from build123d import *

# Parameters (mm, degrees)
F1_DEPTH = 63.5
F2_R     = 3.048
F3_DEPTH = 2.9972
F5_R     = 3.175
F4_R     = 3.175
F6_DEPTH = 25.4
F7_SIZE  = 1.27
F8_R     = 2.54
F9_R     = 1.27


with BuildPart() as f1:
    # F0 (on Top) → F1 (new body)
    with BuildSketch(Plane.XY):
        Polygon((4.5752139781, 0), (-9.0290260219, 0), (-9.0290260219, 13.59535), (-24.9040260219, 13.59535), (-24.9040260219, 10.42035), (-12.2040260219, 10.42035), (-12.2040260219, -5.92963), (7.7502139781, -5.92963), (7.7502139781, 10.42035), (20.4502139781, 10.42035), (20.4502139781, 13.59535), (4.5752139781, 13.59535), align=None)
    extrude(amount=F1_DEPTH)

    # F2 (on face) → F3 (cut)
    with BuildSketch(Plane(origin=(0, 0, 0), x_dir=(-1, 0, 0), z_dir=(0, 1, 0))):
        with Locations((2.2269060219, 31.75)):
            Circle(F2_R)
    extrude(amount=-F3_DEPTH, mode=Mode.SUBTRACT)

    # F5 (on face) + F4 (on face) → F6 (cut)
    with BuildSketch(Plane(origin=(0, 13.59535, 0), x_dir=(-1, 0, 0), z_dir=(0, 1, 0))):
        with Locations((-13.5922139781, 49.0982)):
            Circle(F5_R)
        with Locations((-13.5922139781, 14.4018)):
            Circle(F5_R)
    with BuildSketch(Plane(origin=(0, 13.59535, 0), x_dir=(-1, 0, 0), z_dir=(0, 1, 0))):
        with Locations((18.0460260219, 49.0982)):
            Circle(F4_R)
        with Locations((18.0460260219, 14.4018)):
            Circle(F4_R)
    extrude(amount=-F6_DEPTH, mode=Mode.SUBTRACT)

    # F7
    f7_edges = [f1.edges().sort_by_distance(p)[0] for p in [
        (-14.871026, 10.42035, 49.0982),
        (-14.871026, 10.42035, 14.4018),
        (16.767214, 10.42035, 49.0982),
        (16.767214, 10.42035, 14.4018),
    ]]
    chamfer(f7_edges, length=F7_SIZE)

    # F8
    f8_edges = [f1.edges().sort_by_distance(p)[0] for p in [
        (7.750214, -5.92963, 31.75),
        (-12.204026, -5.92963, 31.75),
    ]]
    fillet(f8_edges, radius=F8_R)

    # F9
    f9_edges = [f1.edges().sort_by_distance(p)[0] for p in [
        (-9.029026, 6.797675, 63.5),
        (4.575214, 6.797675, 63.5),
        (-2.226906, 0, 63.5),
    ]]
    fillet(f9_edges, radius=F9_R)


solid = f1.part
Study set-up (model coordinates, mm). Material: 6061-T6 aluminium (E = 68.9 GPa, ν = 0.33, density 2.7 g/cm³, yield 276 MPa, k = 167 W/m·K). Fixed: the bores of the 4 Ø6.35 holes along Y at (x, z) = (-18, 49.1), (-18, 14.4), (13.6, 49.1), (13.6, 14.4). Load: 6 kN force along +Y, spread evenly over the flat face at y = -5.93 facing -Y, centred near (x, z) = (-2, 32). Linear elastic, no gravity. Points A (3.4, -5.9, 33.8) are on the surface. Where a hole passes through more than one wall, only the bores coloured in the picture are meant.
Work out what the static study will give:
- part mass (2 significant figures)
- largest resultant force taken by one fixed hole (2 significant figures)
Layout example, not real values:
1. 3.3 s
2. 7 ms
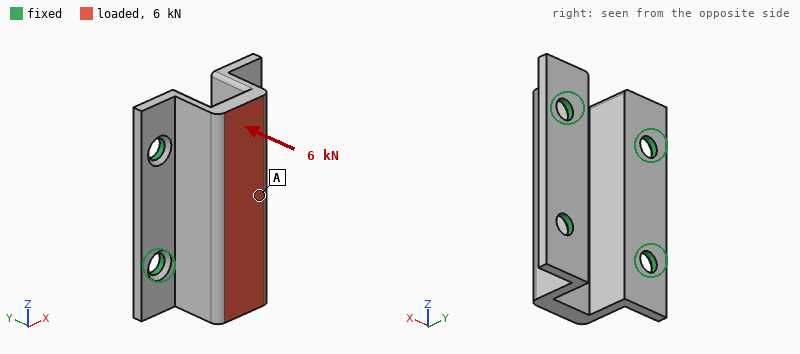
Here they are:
1. 47 g
2. 1.6 kN
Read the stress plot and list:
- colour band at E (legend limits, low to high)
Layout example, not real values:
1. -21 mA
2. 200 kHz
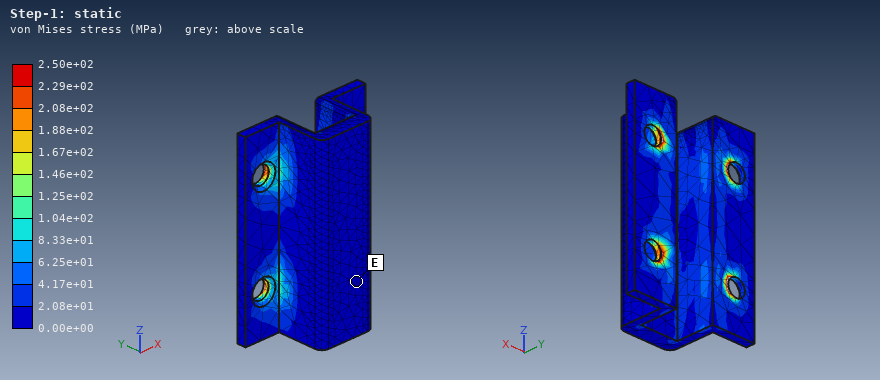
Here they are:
1. 0.00e+00 to 2.08e+01 MPa
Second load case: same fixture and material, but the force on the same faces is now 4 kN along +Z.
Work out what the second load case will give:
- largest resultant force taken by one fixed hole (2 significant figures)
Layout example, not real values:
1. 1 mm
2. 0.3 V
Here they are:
1. 1.5 kN
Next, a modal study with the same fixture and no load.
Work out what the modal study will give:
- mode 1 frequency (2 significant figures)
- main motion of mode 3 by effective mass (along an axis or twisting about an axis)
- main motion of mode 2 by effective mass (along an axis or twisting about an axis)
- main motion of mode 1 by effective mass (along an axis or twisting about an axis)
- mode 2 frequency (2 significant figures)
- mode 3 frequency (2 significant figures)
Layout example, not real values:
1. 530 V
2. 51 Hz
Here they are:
1. 8700 Hz
2. twisting about Y
3. along Z
4. along X
5. 9800 Hz
6. 11 kHz
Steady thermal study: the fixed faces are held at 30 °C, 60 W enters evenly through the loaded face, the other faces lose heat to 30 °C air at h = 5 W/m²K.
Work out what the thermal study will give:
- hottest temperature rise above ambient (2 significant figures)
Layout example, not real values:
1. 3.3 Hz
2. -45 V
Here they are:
1. 23 K
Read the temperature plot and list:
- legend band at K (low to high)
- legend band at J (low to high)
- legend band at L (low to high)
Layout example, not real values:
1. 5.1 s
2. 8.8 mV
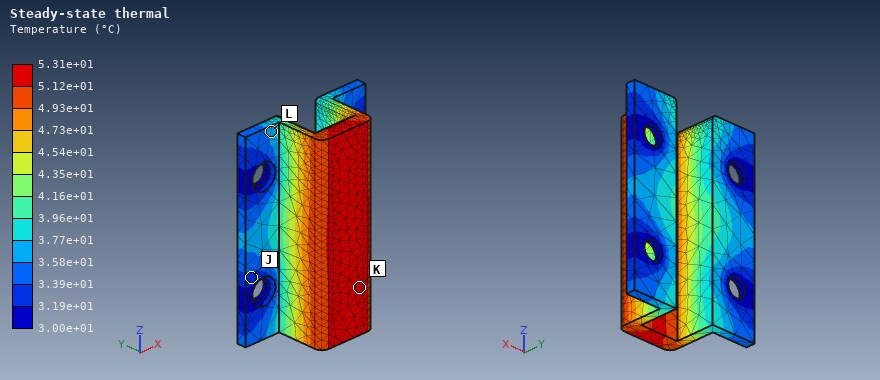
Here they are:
1. 5.12e+01 to 5.31e+01 °C
2. 3.19e+01 to 3.39e+01 °C
3. 3.58e+01 to 3.77e+01 °C
